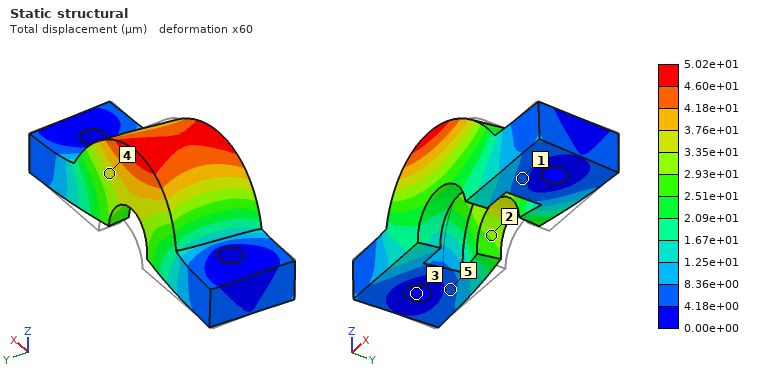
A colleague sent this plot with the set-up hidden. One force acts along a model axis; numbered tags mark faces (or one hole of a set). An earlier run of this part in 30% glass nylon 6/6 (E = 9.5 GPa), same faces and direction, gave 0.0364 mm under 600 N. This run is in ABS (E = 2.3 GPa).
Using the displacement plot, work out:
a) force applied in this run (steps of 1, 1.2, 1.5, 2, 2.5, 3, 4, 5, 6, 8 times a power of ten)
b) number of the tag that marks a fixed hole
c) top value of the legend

200 N
3
5.02e+01 µm
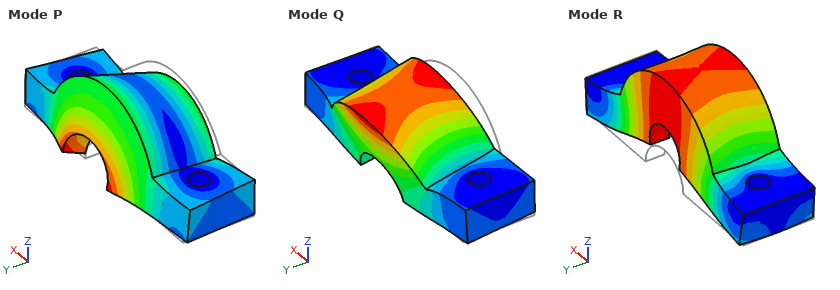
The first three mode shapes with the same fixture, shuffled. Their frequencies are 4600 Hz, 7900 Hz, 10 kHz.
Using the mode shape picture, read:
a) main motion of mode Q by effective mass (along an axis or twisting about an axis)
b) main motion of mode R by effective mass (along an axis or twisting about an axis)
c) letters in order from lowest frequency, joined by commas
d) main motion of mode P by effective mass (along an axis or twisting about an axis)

along Y
along Z
Q, R, P
along Y
